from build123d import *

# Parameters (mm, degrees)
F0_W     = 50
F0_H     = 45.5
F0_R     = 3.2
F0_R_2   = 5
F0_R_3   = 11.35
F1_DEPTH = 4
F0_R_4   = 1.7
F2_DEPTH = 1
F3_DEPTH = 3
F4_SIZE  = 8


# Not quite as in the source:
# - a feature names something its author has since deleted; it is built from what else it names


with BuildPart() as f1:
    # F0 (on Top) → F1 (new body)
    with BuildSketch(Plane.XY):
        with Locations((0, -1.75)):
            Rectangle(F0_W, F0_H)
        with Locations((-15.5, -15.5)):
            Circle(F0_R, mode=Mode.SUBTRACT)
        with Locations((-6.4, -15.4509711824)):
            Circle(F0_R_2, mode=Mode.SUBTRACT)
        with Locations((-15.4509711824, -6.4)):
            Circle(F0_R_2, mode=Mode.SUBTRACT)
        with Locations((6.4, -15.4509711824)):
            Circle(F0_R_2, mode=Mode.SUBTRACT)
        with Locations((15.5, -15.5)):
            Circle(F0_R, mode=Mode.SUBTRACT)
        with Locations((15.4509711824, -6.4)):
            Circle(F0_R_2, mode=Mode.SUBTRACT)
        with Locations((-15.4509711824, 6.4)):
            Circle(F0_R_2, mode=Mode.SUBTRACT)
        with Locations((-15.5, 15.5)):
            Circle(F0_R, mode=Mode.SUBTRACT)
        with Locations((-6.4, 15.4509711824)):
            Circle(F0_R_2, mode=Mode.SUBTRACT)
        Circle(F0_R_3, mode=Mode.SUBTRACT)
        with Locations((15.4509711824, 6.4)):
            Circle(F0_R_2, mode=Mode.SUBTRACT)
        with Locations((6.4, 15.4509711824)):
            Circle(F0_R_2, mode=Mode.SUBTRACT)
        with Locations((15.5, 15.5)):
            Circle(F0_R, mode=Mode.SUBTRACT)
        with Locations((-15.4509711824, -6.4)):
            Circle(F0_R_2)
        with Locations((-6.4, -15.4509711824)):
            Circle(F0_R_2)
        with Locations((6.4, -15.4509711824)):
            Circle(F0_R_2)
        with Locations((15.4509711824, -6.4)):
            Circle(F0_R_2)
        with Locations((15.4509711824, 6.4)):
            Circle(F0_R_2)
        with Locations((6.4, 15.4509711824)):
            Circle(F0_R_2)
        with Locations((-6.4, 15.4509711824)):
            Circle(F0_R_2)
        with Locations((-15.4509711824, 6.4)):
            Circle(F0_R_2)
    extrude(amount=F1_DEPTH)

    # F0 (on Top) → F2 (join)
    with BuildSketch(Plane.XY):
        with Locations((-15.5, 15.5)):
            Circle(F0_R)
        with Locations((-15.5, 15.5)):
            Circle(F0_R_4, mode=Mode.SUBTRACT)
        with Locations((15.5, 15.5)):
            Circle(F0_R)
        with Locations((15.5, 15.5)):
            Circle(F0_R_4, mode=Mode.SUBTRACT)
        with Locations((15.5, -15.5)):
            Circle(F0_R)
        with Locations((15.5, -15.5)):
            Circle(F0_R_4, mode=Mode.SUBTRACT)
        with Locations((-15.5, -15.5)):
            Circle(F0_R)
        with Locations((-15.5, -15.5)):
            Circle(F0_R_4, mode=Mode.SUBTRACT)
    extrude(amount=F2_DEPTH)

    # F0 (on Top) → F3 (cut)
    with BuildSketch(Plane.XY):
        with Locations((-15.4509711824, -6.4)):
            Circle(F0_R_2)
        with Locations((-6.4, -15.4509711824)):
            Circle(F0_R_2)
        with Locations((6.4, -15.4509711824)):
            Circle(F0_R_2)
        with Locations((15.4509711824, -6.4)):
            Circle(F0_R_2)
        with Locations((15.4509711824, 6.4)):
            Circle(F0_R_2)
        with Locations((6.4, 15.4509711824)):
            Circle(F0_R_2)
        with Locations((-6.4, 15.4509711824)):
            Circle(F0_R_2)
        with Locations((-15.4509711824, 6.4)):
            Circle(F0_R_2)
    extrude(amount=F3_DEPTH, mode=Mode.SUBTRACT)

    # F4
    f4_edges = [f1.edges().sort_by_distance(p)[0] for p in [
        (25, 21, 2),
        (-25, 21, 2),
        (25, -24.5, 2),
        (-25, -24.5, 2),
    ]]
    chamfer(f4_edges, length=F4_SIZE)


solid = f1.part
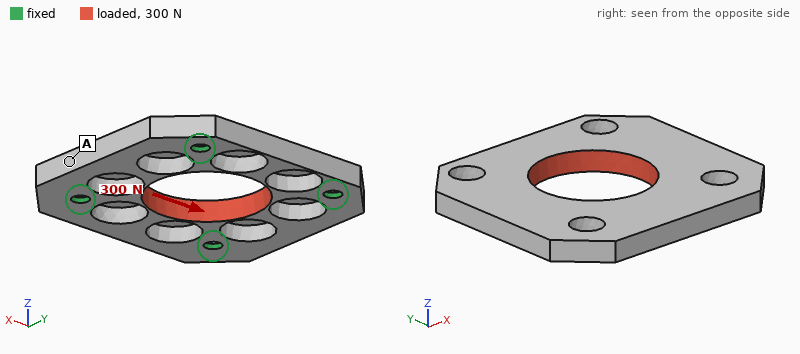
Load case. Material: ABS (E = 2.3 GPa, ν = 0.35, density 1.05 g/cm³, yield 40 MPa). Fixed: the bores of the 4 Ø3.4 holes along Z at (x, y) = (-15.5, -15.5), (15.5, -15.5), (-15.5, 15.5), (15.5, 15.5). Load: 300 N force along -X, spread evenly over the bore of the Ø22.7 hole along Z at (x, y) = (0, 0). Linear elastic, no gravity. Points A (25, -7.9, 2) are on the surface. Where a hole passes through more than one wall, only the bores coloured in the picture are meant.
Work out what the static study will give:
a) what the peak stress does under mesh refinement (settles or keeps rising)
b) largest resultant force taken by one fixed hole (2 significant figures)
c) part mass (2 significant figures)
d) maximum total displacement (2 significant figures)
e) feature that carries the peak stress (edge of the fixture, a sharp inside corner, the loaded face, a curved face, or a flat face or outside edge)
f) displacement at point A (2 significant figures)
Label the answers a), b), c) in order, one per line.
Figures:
a) keeps rising
b) 77 N
c) 4.9 g
d) 88 µm
e) edge of the fixture
f) 71 µm
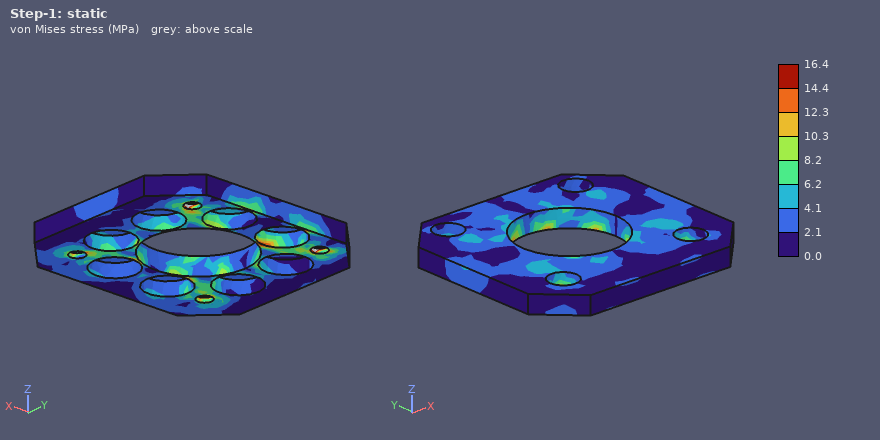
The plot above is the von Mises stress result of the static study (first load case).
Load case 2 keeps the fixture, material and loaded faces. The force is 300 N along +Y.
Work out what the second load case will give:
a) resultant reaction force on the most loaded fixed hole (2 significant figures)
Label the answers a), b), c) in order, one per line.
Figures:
a) 76 N
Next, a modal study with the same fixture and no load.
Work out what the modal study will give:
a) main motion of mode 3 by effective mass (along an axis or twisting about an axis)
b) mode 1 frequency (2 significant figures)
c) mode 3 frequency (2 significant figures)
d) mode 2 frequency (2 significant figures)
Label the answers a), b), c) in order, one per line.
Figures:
a) along Z
b) 2900 Hz
c) 3900 Hz
d) 3200 Hz
